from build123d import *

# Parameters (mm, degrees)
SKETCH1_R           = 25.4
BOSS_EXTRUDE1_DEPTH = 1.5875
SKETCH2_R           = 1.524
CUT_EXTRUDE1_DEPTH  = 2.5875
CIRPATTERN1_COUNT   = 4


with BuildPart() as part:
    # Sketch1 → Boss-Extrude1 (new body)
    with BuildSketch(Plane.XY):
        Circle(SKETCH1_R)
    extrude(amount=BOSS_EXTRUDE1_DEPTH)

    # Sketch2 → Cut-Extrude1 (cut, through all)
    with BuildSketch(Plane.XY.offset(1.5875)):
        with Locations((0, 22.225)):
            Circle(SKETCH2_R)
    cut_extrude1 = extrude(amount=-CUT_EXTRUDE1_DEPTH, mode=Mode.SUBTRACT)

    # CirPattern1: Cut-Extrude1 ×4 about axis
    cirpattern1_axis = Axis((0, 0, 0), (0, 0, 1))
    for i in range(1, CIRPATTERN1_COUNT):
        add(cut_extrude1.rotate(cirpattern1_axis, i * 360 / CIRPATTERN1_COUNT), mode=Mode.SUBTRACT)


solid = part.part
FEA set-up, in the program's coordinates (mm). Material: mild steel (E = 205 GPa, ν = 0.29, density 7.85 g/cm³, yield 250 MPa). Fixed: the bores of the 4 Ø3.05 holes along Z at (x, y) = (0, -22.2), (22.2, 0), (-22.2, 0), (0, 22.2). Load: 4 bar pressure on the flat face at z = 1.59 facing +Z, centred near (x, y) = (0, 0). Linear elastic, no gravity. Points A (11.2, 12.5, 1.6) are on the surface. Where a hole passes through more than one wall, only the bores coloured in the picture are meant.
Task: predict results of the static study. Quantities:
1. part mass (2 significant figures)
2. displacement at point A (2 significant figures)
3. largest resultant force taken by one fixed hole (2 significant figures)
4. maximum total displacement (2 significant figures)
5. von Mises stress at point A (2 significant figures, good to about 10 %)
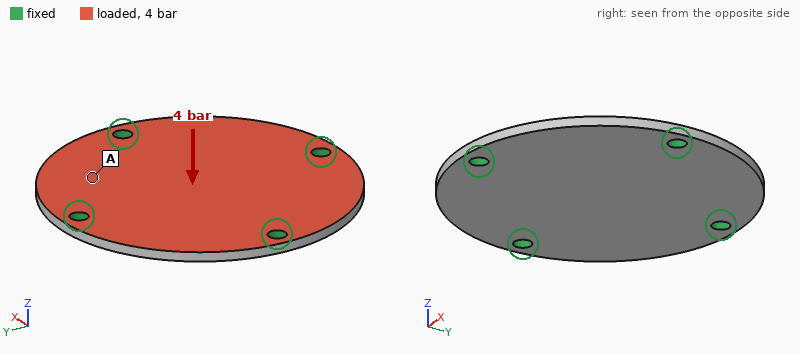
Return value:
25 g
18 µm
200 N
30 µm
46 MPa
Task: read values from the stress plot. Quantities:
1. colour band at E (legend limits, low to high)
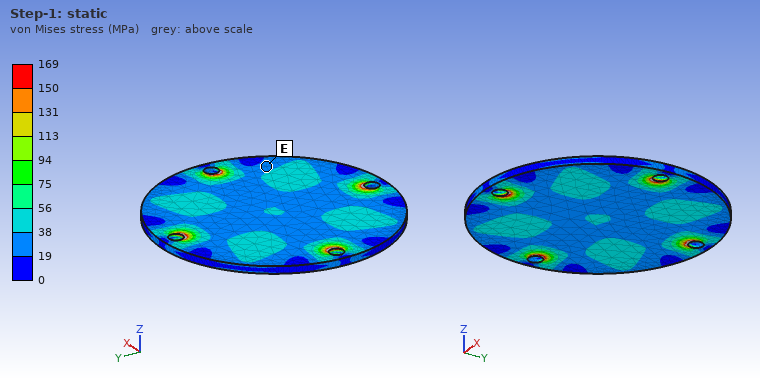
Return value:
19 to 38 MPa
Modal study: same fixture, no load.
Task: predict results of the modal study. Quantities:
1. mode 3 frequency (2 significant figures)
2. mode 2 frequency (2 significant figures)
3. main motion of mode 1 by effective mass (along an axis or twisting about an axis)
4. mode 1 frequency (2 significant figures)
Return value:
7800 Hz
7500 Hz
along Z
6300 Hz
